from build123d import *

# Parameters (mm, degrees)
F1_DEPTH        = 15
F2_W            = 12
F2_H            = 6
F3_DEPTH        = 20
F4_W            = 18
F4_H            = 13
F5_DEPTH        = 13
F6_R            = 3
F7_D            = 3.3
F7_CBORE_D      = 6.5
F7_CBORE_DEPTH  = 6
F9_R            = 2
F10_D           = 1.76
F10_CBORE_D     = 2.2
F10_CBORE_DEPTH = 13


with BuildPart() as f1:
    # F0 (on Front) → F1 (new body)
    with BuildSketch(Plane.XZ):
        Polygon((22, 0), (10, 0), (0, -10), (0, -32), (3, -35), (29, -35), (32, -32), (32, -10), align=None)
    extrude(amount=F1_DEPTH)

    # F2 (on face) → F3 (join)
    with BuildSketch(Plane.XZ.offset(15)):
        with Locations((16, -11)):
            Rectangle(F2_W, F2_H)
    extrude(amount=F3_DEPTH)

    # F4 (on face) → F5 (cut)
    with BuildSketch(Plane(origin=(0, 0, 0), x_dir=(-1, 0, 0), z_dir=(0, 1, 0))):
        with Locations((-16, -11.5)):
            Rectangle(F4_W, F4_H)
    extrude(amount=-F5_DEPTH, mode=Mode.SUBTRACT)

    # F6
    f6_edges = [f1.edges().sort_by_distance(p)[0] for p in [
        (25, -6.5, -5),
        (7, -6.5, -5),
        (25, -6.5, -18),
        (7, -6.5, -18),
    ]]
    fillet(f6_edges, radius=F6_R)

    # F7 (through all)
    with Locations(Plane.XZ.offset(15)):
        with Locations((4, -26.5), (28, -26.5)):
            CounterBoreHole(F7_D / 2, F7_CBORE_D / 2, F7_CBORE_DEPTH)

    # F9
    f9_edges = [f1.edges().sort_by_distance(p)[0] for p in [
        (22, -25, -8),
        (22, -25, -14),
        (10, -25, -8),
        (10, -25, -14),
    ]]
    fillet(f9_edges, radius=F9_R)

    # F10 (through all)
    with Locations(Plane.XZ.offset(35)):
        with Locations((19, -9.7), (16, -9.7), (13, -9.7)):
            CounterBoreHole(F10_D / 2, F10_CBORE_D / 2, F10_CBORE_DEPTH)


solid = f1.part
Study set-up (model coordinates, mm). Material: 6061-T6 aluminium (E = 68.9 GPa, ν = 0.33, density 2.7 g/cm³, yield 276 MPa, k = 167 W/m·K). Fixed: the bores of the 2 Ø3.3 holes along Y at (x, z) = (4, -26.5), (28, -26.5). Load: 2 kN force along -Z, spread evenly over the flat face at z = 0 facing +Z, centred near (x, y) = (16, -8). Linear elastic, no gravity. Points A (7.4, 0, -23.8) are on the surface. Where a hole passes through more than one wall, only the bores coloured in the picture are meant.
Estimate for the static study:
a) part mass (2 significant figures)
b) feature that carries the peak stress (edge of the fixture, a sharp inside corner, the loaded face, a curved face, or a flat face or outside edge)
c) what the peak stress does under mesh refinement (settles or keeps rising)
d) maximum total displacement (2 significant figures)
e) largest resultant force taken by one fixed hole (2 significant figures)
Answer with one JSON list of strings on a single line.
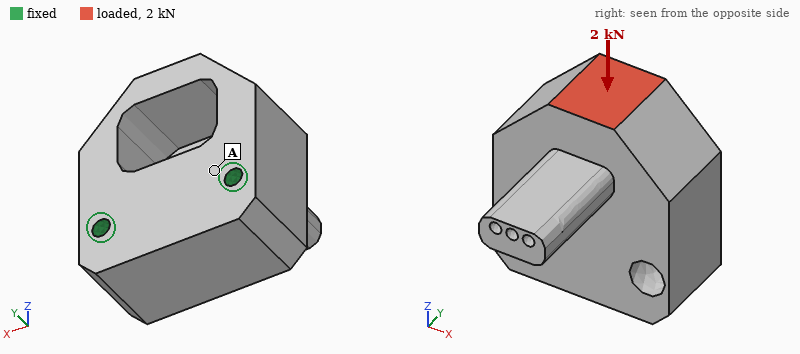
["35 g", "a sharp inside corner", "keeps rising", "22 µm", "1.0 kN"]
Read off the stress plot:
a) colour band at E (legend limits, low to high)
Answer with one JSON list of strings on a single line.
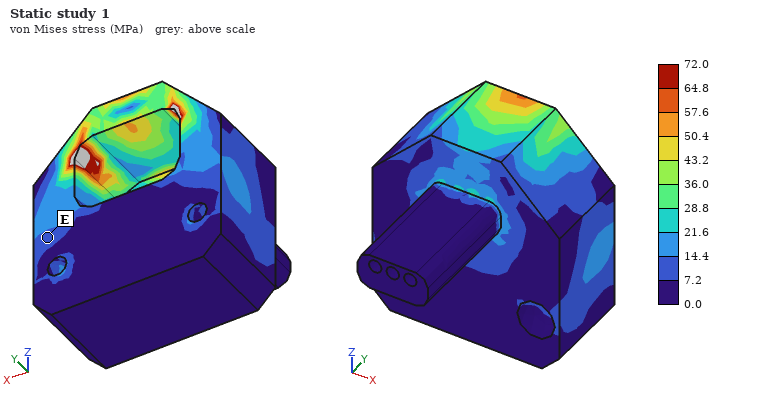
["7.2 to 14.4 MPa"]
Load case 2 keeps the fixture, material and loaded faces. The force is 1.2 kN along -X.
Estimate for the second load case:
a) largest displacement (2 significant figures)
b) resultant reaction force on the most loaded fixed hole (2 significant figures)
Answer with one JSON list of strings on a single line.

["22 µm", "1.4 kN"]
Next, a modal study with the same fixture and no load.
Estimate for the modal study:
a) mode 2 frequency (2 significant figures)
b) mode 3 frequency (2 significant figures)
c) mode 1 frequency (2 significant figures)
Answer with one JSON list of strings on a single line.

["11 kHz", "11 kHz", "6500 Hz"]
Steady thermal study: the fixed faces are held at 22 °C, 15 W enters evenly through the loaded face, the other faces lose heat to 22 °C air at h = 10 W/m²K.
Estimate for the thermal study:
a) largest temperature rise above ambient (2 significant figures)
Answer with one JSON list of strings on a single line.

["15 K"]
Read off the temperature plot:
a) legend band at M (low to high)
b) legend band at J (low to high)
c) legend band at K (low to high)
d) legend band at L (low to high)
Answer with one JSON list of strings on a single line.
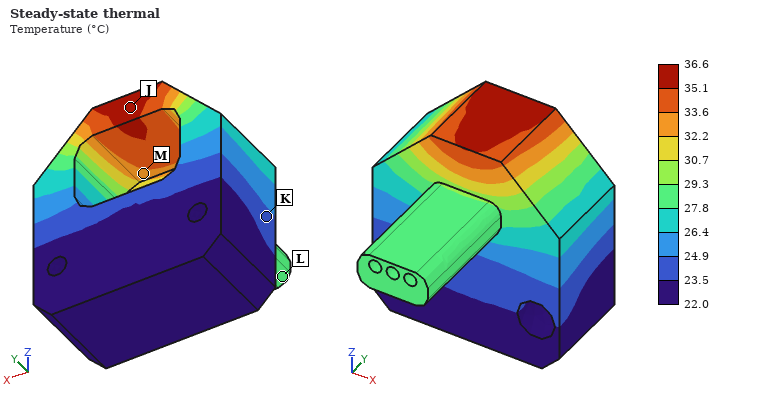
["32.2 to 33.6 °C", "35.1 to 36.6 °C", "23.5 to 24.9 °C", "27.8 to 29.3 °C"]
